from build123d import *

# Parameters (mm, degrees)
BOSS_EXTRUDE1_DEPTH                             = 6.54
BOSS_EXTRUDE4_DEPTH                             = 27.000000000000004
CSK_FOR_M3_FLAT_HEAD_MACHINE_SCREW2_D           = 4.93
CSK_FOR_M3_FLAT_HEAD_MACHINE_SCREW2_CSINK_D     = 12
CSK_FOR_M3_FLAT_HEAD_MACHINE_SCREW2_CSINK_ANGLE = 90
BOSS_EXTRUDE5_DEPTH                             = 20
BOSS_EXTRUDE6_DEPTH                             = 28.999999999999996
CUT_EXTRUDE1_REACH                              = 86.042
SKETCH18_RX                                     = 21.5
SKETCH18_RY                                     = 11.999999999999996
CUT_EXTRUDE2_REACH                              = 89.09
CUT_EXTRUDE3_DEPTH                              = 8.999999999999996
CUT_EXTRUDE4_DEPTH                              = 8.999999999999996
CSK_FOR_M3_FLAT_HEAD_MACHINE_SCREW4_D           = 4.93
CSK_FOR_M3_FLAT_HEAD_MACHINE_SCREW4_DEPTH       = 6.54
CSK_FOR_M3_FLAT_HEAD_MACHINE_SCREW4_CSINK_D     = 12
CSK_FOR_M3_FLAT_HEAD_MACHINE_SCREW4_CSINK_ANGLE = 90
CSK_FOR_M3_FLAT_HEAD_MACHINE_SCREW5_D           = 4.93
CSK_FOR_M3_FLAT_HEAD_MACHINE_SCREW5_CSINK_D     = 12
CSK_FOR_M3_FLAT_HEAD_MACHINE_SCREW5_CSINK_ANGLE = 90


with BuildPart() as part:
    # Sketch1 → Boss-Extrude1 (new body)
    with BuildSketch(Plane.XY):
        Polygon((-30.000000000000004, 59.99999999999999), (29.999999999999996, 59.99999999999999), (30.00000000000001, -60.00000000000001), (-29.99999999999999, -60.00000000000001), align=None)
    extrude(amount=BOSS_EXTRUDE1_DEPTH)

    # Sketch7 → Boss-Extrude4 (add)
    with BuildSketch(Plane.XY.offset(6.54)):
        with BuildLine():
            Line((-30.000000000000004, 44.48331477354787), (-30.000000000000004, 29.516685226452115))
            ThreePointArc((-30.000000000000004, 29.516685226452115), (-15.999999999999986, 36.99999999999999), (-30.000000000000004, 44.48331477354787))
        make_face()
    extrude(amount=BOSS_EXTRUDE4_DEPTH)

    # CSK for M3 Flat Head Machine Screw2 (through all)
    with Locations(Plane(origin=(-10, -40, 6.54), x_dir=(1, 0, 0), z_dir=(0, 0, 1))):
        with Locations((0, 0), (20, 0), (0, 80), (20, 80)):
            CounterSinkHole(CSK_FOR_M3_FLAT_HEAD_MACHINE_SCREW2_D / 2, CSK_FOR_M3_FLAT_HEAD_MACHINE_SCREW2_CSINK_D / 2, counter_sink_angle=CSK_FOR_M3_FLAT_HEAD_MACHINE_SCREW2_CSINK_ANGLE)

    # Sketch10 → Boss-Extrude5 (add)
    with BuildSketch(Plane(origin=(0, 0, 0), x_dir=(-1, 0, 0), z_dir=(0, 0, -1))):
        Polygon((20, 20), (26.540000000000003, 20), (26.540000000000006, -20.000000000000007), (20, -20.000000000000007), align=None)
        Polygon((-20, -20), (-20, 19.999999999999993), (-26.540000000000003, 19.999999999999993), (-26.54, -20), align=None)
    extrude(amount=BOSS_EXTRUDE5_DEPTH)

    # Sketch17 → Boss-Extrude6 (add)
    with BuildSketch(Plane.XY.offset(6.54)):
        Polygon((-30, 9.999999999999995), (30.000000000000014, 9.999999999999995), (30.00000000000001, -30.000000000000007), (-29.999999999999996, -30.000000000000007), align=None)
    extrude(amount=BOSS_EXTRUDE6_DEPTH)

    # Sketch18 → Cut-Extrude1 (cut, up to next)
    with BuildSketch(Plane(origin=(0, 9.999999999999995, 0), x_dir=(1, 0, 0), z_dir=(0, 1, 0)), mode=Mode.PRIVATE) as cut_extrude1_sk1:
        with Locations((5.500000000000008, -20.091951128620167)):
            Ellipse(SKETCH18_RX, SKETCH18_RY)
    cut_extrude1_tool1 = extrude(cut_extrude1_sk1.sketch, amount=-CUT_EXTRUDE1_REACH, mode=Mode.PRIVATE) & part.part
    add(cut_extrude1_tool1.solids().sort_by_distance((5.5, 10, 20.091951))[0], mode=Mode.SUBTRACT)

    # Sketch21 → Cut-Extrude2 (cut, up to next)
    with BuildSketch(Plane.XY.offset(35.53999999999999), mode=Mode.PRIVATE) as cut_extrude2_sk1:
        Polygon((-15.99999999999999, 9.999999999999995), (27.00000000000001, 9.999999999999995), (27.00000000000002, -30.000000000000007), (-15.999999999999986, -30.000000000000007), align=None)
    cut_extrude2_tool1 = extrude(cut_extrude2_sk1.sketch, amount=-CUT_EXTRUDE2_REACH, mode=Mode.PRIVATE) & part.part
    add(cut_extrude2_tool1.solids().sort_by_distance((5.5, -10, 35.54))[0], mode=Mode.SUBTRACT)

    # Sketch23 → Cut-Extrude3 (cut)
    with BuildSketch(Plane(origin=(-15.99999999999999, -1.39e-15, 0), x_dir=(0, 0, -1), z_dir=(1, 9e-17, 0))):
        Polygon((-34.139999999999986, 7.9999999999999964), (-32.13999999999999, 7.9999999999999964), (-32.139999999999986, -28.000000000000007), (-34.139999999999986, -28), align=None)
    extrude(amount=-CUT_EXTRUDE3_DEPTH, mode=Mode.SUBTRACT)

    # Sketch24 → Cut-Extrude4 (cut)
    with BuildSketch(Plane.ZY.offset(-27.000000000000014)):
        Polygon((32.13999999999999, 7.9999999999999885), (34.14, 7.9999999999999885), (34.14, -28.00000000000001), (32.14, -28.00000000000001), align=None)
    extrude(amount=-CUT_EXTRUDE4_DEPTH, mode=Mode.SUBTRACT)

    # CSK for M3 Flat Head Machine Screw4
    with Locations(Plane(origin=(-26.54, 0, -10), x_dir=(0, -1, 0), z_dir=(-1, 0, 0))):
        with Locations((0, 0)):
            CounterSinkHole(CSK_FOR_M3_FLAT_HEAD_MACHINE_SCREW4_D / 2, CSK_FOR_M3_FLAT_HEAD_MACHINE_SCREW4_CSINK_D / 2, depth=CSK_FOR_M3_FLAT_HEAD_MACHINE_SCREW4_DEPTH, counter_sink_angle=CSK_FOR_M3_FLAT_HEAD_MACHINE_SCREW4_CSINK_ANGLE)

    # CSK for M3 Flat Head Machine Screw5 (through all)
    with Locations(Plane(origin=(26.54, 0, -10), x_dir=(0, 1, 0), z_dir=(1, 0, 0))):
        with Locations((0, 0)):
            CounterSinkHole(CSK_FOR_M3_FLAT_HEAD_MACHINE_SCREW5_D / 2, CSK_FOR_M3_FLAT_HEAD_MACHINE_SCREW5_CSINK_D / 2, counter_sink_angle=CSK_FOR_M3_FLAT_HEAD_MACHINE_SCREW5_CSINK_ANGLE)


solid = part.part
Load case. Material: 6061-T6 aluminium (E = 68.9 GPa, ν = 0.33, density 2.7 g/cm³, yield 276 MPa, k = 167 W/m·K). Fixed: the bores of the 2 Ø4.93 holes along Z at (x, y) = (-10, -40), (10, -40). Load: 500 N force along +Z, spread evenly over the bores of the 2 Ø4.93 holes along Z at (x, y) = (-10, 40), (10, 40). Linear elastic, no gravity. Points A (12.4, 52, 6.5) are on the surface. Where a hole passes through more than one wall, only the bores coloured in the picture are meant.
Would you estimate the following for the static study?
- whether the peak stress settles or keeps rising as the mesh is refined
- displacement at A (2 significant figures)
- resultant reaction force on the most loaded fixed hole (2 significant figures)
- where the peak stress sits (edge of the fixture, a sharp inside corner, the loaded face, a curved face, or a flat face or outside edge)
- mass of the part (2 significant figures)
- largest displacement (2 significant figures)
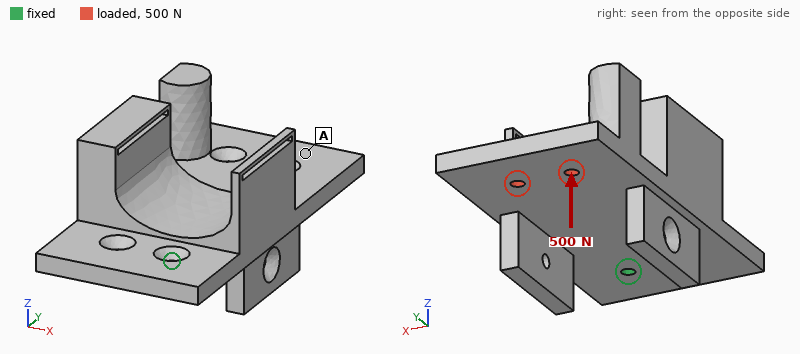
keeps rising
1.00 mm
360 N
edge of the fixture
240 g
1.1 mm
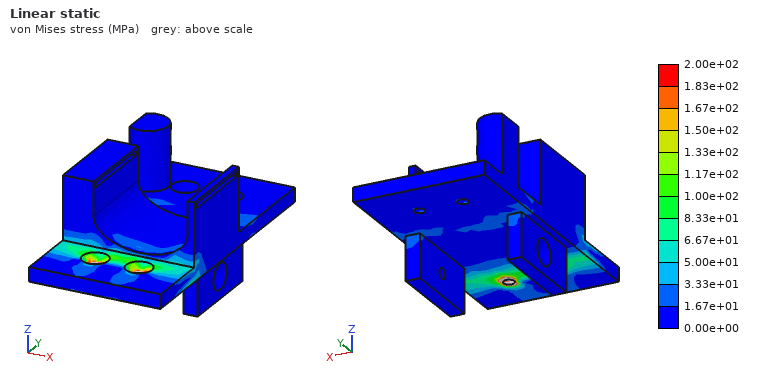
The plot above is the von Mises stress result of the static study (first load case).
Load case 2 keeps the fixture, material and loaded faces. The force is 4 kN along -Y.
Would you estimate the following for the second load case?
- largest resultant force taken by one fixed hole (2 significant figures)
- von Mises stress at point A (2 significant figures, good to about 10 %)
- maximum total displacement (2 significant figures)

2.0 kN
7.9 MPa
0.18 mm
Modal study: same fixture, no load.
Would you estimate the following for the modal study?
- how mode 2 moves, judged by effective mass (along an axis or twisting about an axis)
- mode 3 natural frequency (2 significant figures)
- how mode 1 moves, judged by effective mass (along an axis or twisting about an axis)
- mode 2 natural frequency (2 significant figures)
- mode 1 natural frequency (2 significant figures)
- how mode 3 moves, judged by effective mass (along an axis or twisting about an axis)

twisting about Y
1900 Hz
along Z
1500 Hz
410 Hz
along X
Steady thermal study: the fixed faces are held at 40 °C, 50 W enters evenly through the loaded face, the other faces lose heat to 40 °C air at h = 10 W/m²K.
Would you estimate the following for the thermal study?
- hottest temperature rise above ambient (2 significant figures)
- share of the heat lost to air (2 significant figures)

55 K
13 %
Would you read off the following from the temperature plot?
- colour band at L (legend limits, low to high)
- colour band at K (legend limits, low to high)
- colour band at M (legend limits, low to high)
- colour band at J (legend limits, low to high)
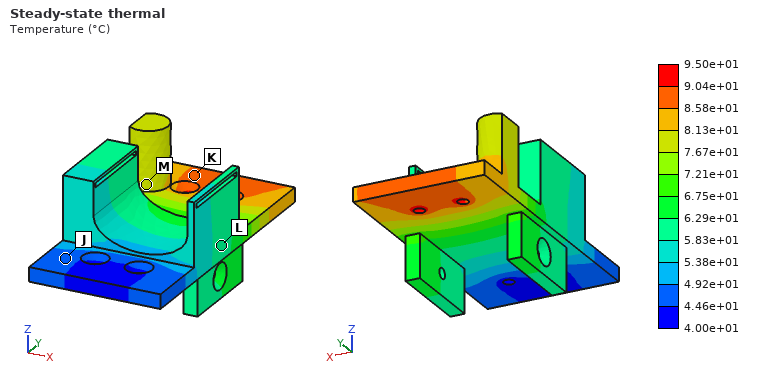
5.83e+01 to 6.29e+01 °C
8.58e+01 to 9.04e+01 °C
7.67e+01 to 8.13e+01 °C
4.46e+01 to 4.92e+01 °C
